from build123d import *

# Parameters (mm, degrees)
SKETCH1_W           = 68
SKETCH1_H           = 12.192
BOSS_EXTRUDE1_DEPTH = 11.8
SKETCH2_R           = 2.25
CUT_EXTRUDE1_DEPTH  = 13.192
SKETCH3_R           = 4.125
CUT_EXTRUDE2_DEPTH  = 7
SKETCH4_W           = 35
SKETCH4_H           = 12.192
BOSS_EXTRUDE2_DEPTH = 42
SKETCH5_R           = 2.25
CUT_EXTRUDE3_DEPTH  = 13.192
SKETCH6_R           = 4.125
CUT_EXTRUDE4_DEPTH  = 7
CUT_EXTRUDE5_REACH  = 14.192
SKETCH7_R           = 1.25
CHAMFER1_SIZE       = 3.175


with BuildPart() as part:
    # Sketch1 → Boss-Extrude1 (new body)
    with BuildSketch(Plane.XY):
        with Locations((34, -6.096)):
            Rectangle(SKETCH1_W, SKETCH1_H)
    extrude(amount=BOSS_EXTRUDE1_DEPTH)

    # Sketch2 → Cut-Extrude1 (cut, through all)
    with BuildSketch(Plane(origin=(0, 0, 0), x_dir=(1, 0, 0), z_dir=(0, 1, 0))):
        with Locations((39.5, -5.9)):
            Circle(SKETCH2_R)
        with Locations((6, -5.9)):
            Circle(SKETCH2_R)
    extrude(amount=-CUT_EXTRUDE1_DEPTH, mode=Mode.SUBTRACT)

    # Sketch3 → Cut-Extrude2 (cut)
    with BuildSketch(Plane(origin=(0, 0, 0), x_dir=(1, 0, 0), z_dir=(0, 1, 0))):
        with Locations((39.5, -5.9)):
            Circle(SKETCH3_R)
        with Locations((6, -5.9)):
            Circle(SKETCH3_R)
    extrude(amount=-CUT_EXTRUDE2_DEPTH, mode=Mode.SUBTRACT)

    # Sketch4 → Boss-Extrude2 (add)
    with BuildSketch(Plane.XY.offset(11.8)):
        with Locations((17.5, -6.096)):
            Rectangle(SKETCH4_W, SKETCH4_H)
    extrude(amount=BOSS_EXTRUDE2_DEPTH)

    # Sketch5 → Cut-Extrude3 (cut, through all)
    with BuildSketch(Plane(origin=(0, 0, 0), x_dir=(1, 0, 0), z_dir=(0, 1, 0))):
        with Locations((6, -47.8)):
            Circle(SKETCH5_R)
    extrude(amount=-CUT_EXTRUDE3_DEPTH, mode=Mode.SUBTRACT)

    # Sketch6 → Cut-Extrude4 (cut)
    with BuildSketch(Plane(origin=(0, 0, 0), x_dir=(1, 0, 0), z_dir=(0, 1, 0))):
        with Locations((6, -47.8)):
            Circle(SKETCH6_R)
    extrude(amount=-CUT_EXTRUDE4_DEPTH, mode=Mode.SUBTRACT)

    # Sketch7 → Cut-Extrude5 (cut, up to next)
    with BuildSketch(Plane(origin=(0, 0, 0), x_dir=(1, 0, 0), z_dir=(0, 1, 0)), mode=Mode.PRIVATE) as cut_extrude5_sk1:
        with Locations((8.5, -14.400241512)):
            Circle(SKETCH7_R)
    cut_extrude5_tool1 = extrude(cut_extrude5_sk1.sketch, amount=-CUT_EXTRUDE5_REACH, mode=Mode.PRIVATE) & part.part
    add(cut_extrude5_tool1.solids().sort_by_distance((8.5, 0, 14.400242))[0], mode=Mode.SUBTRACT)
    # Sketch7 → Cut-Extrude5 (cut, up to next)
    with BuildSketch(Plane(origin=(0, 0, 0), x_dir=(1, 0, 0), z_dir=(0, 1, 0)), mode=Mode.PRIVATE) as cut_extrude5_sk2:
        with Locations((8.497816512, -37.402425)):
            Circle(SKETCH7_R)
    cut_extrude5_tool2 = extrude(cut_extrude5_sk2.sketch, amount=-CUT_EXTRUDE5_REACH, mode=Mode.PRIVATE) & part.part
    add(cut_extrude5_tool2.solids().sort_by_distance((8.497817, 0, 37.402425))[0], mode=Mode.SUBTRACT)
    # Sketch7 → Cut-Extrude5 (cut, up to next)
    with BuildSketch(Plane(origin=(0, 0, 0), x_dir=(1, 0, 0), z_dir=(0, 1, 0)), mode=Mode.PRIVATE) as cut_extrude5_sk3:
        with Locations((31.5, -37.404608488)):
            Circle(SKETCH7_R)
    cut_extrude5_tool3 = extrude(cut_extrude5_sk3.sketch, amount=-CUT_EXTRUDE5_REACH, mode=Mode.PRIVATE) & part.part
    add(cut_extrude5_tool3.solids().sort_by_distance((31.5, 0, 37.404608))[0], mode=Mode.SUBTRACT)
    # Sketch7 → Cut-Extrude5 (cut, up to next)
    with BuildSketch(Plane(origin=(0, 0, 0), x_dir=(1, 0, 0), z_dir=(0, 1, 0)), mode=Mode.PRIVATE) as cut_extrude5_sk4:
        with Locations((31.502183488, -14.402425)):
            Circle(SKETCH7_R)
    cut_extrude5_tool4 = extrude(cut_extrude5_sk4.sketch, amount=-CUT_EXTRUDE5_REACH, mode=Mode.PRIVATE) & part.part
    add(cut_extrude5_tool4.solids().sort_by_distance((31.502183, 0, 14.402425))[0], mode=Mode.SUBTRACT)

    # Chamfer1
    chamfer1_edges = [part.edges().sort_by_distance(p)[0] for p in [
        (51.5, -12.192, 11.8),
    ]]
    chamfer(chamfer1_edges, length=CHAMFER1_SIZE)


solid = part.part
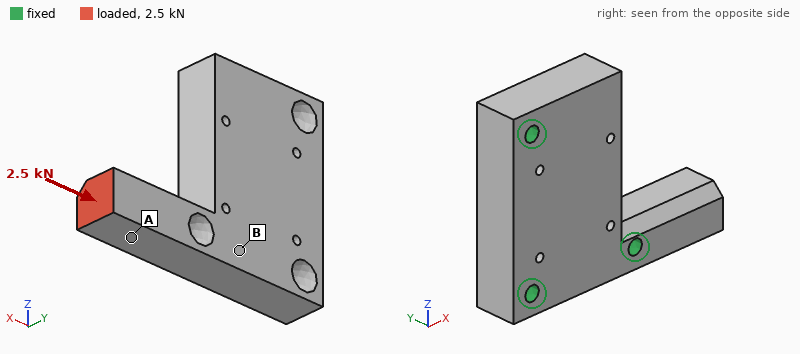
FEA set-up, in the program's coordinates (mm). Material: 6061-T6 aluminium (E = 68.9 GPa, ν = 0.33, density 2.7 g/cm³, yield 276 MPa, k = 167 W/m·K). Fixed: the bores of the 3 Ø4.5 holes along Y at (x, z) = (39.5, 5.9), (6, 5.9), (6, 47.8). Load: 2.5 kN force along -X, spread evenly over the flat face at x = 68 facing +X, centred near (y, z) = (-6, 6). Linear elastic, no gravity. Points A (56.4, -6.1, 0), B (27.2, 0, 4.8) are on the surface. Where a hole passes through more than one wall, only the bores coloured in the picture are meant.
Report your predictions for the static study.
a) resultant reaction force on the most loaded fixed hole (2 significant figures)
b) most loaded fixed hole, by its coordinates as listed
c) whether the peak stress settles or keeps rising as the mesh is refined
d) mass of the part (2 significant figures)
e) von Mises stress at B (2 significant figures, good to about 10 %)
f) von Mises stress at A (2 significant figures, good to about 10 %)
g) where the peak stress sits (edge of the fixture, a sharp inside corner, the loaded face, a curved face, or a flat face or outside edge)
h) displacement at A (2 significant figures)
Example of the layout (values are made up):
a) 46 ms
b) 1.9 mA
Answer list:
a) 2.0 kN
b) (39.5, 5.9)
c) keeps rising
d) 70 g
e) 7.2 MPa
f) 18 MPa
g) edge of the fixture
h) 16 µm
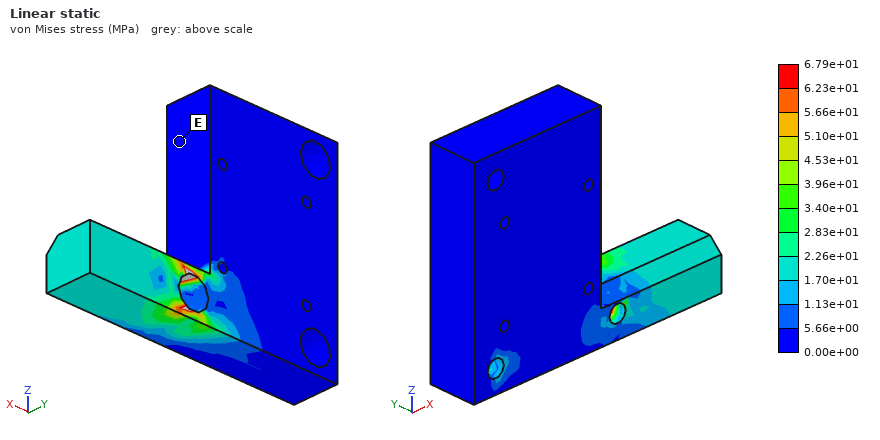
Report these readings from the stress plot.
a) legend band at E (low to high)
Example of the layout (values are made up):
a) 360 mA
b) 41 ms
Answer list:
a) 0.00e+00 to 5.66e+00 MPa
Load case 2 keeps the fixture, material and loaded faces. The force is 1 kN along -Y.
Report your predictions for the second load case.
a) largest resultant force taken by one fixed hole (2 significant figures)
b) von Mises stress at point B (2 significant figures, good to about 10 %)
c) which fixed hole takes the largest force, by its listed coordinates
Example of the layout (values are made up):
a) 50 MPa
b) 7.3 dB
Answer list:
a) 1.9 kN
b) 19 MPa
c) (39.5, 5.9)
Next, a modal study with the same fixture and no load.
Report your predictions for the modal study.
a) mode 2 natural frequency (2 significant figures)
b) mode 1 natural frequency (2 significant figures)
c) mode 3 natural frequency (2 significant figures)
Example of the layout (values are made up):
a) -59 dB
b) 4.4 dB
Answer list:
a) 8000 Hz
b) 7400 Hz
c) 8200 Hz
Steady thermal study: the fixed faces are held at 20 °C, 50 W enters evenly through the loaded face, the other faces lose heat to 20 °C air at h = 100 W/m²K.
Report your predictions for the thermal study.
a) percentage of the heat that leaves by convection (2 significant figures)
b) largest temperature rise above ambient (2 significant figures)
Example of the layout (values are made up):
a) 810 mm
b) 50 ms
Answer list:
a) 11 %
b) 65 K
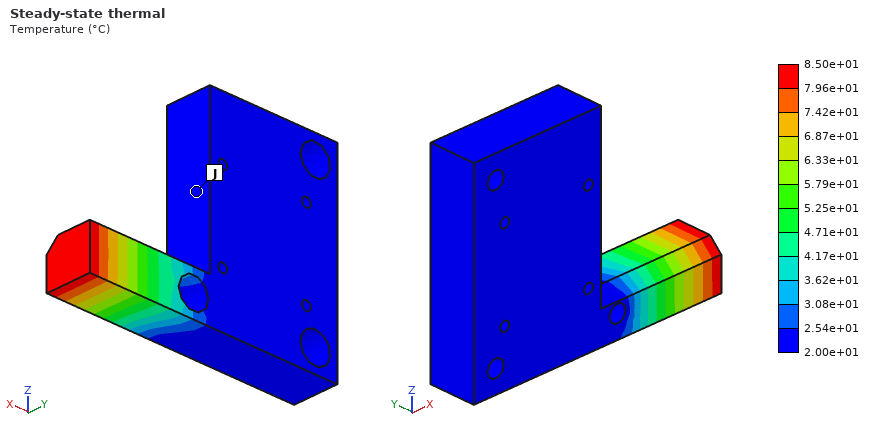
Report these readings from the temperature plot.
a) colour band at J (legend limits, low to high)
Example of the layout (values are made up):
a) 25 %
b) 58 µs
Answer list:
a) 2.00e+01 to 2.54e+01 °C
